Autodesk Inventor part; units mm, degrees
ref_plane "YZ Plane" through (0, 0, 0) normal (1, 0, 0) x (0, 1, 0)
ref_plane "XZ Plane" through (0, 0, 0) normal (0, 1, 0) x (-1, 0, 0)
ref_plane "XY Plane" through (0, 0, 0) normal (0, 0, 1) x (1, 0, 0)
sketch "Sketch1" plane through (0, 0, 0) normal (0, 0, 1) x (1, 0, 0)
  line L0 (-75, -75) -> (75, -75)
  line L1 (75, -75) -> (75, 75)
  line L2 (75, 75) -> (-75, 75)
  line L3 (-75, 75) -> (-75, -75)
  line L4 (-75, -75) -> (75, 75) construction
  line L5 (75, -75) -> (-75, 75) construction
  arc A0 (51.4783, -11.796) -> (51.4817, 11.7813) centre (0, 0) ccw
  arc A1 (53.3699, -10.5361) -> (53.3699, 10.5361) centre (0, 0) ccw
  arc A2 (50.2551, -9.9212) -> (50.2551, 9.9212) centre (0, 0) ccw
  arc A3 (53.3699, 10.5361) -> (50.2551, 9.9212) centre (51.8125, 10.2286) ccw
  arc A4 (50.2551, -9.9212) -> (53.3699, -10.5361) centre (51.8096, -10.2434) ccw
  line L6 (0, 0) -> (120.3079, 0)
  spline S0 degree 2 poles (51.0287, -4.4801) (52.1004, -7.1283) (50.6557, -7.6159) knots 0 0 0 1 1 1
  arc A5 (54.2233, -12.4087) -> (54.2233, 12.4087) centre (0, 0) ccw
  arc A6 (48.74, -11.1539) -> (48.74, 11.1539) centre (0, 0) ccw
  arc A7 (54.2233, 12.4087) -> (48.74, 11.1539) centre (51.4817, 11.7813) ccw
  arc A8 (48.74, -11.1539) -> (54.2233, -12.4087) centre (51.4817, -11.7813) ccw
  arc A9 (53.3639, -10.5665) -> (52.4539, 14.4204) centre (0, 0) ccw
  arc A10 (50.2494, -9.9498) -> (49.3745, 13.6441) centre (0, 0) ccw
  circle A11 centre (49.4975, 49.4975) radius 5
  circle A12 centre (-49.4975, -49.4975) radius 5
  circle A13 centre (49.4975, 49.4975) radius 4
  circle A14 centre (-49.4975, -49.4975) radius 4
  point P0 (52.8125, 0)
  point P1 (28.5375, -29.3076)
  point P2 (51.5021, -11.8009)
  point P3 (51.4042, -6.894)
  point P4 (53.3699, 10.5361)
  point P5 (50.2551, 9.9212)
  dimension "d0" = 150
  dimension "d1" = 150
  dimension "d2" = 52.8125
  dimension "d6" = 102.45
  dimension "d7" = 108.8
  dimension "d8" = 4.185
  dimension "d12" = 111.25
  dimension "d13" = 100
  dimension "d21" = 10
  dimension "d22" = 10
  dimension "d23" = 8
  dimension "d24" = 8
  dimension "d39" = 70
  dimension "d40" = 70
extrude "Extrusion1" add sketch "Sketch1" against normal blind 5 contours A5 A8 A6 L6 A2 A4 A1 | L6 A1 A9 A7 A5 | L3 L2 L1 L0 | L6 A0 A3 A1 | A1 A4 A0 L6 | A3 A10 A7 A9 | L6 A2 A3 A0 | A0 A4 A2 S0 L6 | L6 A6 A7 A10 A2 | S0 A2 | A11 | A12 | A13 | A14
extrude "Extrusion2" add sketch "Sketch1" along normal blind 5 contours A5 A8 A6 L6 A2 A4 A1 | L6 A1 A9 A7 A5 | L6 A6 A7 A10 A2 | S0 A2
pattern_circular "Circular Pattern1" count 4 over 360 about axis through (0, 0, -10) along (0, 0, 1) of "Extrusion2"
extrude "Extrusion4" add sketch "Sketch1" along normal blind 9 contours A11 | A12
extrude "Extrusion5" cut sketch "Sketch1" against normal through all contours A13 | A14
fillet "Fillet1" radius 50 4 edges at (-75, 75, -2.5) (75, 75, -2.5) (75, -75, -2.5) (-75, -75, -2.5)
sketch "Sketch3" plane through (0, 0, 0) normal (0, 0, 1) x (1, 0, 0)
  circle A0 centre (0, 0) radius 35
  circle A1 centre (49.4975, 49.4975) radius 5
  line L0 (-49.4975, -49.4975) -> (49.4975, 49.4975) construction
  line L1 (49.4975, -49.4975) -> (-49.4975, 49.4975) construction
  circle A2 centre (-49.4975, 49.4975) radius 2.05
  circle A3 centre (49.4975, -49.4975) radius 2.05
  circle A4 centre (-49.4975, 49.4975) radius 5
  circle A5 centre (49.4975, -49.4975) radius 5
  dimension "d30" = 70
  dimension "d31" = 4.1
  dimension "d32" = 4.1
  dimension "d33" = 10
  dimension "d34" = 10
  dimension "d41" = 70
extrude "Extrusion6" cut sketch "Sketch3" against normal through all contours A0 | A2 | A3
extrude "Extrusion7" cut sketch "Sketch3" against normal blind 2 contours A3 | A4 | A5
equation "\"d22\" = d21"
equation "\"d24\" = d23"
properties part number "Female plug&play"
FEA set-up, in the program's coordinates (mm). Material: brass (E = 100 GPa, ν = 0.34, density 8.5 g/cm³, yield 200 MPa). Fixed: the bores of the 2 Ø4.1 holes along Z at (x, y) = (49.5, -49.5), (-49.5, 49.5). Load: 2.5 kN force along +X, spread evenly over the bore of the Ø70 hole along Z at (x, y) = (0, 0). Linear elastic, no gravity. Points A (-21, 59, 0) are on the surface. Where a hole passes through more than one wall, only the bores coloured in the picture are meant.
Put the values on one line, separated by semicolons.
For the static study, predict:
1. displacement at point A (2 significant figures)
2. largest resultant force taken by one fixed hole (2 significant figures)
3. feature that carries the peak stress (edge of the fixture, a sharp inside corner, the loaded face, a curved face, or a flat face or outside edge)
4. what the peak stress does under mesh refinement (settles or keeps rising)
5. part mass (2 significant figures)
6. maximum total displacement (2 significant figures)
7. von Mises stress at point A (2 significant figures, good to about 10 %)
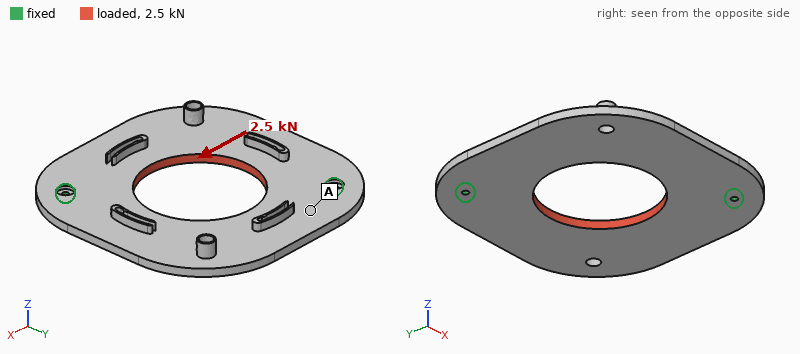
12 µm; 1.3 kN; edge of the fixture; keeps rising; 710 g; 32 µm; 3.9 MPa
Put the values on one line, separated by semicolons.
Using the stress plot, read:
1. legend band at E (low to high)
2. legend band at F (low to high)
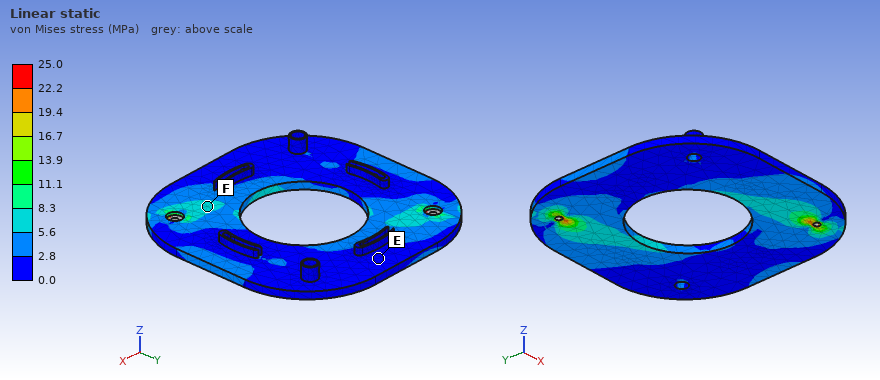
0.0 to 2.8 MPa; 5.6 to 8.3 MPa
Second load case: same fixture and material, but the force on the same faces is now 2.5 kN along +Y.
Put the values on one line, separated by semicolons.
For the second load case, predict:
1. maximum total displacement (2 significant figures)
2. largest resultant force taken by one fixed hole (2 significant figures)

32 µm; 1.3 kN
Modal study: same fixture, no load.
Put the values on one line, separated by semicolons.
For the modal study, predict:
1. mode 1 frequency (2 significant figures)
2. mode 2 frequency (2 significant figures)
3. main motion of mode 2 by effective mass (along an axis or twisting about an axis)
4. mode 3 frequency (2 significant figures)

240 Hz; 350 Hz; along Z; 860 Hz
